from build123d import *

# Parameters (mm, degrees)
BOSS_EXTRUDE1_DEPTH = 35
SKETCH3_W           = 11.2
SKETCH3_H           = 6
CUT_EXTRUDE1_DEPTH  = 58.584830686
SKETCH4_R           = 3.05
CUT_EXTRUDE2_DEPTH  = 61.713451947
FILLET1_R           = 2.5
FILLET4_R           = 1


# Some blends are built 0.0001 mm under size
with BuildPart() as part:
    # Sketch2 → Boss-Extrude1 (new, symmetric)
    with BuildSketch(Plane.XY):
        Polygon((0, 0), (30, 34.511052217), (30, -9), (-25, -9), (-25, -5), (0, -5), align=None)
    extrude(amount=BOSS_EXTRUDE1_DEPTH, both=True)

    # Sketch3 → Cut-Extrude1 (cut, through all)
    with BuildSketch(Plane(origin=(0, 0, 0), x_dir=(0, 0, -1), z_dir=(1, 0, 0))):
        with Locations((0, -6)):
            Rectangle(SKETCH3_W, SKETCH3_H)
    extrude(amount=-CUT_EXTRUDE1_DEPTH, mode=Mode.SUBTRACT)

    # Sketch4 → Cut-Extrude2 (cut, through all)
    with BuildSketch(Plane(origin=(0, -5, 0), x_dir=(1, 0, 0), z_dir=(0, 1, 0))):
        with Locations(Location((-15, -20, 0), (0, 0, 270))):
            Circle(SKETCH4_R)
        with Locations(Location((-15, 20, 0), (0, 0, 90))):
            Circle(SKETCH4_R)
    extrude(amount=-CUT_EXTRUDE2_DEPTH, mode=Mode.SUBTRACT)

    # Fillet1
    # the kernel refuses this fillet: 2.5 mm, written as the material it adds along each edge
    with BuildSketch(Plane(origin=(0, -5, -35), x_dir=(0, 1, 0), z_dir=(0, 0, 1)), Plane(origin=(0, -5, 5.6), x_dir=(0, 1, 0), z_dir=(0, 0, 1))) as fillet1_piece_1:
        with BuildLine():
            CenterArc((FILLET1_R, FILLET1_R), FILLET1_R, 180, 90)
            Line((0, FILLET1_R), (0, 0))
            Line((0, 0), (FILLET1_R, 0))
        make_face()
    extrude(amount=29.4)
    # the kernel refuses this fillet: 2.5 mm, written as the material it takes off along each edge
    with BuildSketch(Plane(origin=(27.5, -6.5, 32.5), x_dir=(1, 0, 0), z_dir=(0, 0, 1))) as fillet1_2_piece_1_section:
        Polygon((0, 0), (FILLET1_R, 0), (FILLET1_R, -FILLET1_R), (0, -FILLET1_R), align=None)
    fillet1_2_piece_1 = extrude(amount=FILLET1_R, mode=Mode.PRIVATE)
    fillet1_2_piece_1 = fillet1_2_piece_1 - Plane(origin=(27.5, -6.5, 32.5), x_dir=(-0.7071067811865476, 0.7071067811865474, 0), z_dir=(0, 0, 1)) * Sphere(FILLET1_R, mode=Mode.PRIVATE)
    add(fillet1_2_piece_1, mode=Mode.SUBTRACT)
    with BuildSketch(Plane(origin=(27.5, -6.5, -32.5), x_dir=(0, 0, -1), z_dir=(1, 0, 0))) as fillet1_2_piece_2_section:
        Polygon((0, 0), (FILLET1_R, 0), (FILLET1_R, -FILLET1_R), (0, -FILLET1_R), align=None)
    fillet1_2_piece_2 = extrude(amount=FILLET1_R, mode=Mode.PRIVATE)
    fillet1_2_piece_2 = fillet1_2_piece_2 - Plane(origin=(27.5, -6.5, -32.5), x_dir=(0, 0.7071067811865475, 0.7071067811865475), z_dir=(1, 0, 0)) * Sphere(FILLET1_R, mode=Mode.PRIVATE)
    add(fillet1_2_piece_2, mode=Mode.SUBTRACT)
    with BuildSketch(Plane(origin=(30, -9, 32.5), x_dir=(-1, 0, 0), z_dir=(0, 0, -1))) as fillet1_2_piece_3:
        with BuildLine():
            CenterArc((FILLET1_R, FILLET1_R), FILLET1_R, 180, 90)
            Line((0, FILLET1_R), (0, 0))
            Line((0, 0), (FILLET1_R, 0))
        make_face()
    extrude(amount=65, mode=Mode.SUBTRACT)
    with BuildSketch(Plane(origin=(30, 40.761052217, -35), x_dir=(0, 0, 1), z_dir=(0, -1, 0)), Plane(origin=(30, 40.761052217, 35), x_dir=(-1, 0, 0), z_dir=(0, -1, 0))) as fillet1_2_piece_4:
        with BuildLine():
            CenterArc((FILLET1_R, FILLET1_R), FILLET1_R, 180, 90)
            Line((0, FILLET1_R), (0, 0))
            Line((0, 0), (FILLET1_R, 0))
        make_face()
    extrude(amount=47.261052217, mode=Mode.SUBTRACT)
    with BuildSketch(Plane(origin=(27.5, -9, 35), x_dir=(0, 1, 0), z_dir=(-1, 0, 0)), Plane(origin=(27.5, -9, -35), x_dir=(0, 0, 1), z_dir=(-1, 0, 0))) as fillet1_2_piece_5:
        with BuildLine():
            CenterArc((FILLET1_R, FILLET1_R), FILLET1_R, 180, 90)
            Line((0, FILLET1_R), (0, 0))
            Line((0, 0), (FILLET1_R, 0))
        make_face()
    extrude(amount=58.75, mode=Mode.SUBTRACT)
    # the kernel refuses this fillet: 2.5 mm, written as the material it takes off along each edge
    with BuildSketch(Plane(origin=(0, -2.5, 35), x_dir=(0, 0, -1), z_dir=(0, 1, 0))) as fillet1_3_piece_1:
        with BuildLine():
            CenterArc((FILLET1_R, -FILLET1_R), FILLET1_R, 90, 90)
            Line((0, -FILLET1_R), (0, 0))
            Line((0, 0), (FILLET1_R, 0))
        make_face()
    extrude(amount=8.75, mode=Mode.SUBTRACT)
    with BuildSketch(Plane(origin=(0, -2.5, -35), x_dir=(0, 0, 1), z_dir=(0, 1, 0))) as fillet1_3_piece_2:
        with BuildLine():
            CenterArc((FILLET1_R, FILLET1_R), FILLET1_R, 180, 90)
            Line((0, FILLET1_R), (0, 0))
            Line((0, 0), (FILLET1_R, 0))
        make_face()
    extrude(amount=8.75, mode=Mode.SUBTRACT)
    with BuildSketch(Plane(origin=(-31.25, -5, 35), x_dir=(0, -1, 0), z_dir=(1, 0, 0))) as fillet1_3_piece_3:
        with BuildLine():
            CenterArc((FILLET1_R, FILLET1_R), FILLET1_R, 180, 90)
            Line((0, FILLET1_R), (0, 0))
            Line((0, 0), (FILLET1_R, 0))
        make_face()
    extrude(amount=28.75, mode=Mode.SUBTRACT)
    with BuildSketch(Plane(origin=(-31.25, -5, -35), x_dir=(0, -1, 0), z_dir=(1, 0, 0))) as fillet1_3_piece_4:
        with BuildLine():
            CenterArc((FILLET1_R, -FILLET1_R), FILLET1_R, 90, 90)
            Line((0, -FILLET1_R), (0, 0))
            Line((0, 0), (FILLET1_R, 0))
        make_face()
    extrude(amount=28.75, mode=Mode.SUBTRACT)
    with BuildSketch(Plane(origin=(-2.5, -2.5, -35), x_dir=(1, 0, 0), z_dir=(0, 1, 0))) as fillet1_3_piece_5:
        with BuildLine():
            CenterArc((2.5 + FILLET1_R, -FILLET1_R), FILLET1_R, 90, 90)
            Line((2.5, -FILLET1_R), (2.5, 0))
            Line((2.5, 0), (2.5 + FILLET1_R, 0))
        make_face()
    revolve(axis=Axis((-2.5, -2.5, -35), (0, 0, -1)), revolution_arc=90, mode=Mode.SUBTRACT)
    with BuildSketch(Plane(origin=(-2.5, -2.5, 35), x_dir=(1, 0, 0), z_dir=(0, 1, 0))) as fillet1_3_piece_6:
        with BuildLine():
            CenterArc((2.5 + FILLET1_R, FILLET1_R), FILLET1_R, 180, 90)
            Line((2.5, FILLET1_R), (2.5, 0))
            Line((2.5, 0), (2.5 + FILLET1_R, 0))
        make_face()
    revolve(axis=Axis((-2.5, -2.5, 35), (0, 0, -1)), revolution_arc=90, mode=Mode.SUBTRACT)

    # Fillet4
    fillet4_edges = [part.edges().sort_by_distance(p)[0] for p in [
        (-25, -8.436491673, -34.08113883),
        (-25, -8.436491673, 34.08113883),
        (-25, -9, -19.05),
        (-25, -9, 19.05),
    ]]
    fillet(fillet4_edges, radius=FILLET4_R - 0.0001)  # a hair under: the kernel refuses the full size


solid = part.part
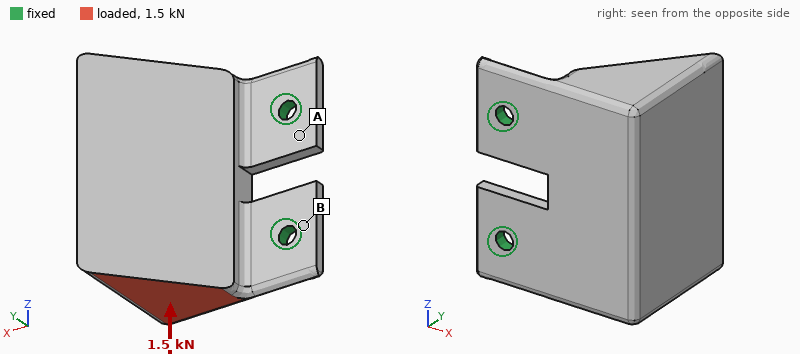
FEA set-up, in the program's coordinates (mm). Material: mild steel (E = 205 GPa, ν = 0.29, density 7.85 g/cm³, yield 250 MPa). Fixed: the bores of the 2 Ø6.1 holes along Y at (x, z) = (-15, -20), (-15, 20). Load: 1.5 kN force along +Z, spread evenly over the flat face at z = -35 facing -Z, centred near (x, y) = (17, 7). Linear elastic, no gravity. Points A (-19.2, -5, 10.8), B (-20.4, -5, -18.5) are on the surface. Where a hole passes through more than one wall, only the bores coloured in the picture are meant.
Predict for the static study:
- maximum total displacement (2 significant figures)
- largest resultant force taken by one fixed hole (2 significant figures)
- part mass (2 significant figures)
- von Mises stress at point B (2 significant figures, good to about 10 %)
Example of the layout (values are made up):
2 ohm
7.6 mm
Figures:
20 µm
1.3 kN
470 g
10 MPa
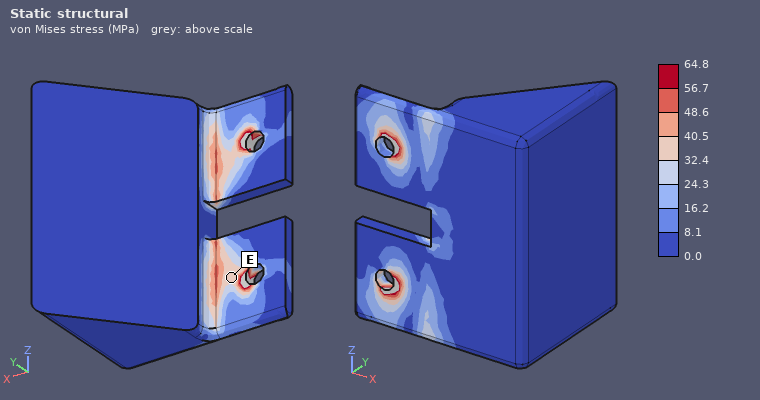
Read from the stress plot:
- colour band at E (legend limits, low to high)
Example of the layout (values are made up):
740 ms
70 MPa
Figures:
32.4 to 40.5 MPa
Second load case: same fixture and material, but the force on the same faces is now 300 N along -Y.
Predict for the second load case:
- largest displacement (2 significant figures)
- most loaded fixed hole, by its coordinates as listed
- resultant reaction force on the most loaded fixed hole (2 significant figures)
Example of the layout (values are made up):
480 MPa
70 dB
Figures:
0.10 mm
(-15, -20)
380 N
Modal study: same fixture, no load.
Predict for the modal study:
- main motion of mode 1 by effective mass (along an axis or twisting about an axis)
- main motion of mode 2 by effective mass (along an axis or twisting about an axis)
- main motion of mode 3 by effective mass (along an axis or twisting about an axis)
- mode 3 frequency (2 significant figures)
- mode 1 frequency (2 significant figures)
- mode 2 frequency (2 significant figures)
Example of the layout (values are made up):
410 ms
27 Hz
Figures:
along Y
along Z
along Z
4600 Hz
500 Hz
2300 Hz
